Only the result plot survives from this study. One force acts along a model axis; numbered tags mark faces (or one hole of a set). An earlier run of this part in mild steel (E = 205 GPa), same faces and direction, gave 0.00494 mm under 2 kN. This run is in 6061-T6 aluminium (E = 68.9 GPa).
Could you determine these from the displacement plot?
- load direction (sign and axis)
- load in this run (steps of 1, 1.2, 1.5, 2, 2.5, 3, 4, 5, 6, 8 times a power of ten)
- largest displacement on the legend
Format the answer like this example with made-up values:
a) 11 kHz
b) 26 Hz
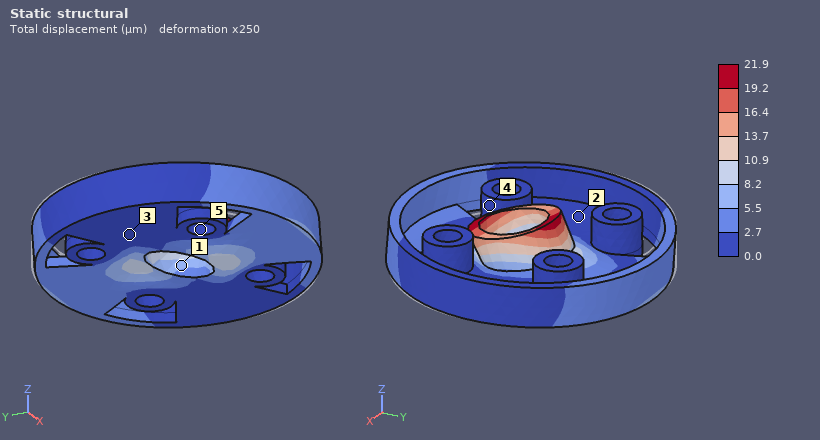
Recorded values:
a) -Y
b) 3 kN
c) 21.9 µm
